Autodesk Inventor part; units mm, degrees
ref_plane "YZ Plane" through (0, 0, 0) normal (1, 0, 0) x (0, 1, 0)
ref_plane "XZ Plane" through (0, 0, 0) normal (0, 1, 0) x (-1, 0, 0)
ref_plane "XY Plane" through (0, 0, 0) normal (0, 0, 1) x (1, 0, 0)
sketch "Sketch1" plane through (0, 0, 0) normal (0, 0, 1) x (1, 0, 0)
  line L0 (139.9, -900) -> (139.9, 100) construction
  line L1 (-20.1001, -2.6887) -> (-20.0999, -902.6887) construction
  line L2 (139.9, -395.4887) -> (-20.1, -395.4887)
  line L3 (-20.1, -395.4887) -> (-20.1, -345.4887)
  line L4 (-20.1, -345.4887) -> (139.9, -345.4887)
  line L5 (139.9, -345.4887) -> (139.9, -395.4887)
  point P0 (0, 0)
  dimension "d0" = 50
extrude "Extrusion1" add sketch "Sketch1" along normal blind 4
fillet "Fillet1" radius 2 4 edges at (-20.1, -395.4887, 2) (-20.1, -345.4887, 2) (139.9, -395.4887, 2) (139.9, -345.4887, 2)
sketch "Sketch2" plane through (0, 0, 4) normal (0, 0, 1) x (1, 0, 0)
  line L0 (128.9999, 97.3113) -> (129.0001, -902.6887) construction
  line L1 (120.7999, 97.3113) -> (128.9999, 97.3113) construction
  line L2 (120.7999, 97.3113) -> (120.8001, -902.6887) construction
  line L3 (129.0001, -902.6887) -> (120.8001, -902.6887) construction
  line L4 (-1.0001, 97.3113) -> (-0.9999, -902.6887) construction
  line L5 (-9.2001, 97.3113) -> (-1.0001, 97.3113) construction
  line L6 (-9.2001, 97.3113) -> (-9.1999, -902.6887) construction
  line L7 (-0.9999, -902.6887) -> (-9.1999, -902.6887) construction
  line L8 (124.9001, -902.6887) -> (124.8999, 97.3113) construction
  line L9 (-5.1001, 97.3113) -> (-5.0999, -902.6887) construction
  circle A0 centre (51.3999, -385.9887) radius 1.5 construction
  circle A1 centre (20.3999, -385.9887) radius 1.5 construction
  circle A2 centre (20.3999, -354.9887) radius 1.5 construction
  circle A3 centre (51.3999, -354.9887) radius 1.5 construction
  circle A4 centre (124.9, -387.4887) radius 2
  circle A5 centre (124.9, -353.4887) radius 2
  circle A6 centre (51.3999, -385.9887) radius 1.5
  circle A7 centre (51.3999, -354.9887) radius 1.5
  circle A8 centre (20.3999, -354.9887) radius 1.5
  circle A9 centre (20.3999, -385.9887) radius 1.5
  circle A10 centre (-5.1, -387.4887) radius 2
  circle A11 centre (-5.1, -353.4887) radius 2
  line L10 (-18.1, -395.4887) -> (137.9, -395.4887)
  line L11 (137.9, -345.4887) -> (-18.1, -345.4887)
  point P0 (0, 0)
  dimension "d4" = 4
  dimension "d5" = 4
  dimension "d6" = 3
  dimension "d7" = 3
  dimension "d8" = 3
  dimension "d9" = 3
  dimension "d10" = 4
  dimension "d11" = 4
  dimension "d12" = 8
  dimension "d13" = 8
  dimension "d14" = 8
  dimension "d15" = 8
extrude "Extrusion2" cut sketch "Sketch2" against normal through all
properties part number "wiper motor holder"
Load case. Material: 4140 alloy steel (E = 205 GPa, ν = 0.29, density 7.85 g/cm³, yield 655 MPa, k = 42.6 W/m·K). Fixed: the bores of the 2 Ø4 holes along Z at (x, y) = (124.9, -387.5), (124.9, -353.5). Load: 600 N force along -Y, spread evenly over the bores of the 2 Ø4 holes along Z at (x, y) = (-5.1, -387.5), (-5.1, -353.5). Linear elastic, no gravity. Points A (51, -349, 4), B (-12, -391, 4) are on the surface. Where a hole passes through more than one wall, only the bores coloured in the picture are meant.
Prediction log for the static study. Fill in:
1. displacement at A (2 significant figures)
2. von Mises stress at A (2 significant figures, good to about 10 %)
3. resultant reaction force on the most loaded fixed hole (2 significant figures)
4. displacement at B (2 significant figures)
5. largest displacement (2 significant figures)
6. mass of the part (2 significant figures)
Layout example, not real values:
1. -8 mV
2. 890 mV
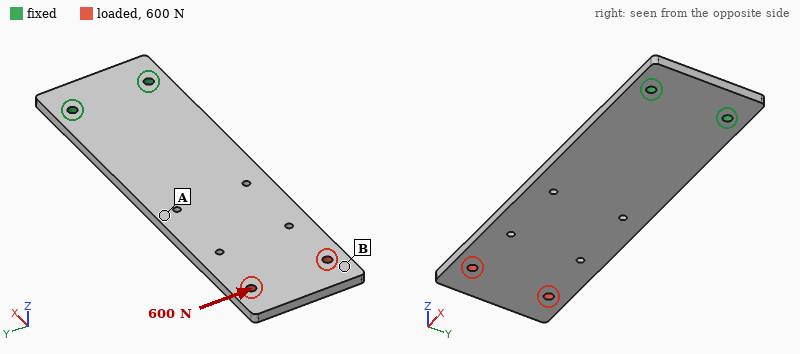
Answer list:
1. 28 µm
2. 18 MPa
3. 2.2 kN
4. 67 µm
5. 72 µm
6. 250 g
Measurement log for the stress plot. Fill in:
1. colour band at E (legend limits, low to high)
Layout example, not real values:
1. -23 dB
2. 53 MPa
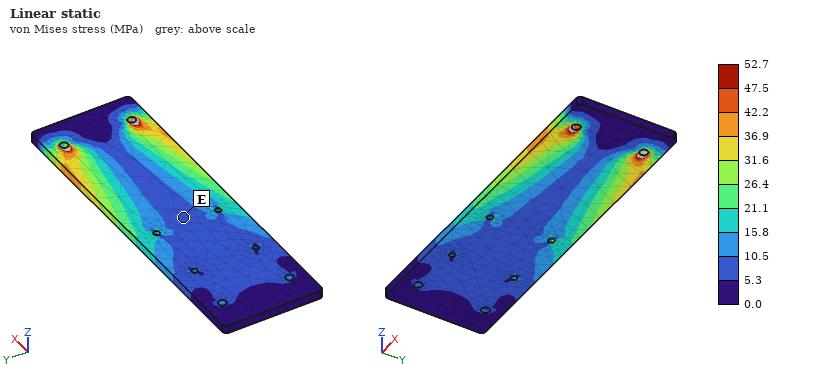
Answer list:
1. 5.3 to 10.5 MPa
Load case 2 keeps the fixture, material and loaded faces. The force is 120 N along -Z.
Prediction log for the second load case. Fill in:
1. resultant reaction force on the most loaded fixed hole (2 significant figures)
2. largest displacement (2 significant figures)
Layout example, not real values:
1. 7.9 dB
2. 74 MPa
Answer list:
1. 60 N
2. 1.9 mm
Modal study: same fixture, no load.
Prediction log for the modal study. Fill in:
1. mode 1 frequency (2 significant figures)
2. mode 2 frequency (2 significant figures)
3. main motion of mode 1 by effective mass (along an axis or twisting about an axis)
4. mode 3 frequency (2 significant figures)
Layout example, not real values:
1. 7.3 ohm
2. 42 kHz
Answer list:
1. 160 Hz
2. 940 Hz
3. along Z
4. 970 Hz
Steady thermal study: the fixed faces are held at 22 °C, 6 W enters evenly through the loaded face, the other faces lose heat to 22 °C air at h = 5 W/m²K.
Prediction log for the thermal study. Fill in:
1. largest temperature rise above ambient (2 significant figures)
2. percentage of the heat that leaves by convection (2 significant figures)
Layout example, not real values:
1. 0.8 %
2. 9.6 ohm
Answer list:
1. 67 K
2. 44 %
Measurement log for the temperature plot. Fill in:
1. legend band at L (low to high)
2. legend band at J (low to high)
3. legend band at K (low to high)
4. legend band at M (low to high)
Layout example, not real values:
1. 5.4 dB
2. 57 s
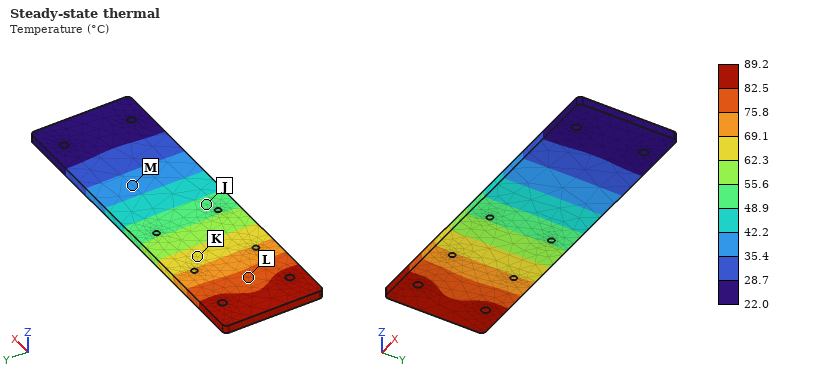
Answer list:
1. 75.8 to 82.5 °C
2. 48.9 to 55.6 °C
3. 62.3 to 69.1 °C
4. 35.4 to 42.2 °C
